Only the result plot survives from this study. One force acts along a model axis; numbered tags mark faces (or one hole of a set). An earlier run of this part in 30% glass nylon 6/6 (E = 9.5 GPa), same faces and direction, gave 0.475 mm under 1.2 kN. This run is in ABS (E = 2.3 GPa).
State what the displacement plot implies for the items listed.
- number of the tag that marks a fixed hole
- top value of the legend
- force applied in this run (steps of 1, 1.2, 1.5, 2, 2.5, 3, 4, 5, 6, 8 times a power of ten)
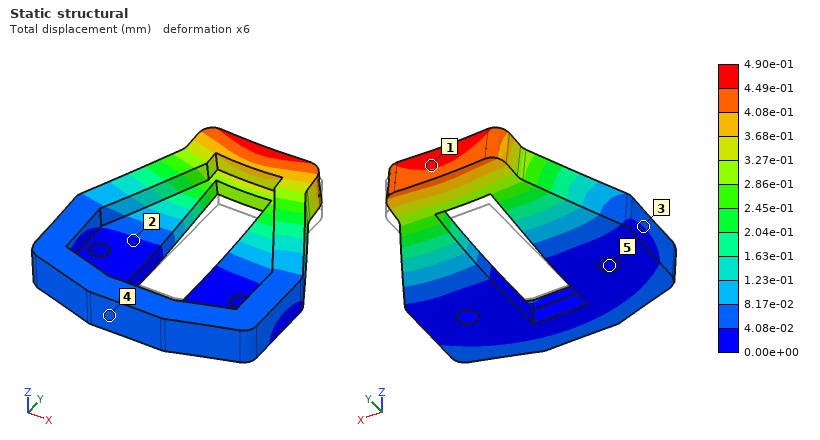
5
4.90e-01 mm
300 N
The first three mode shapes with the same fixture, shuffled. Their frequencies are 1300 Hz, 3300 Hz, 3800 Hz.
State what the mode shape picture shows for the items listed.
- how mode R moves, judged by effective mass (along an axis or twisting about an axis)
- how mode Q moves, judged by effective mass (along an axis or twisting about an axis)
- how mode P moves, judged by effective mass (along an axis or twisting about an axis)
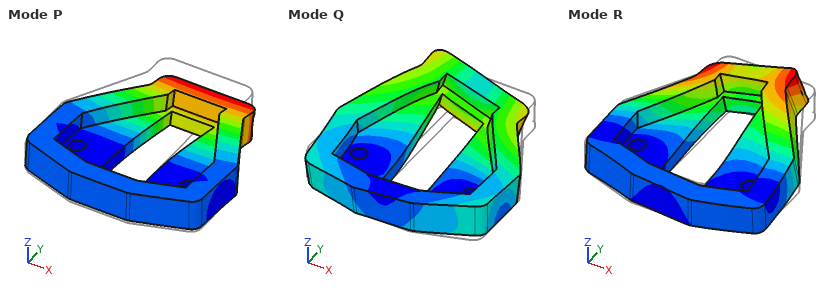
along X
along X
along Z
